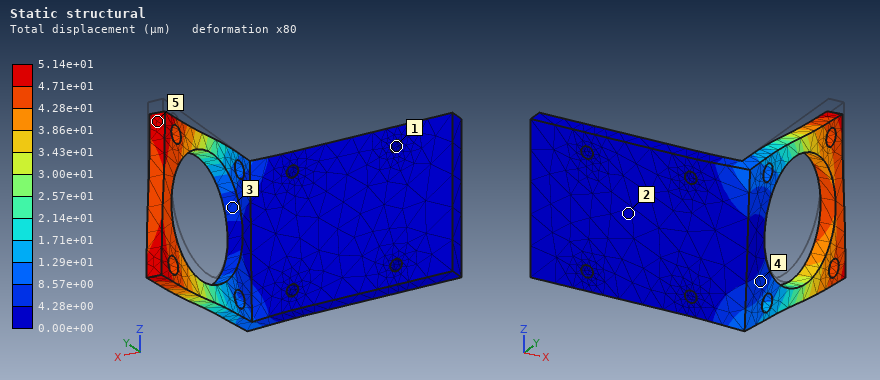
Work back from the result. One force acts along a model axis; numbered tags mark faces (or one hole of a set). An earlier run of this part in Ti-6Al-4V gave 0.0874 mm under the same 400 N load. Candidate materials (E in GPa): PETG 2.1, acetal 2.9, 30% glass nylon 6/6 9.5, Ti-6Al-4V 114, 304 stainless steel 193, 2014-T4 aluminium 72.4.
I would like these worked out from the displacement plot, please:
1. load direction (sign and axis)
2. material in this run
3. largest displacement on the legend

-Z
304 stainless steel
5.14e+01 µm
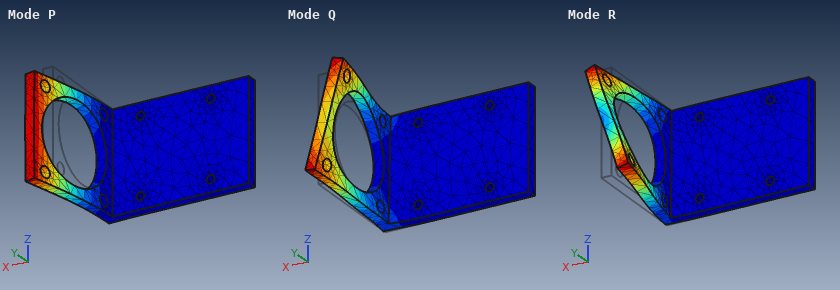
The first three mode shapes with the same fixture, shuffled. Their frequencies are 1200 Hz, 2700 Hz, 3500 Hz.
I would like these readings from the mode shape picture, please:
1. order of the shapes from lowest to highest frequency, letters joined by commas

P, R, Q
